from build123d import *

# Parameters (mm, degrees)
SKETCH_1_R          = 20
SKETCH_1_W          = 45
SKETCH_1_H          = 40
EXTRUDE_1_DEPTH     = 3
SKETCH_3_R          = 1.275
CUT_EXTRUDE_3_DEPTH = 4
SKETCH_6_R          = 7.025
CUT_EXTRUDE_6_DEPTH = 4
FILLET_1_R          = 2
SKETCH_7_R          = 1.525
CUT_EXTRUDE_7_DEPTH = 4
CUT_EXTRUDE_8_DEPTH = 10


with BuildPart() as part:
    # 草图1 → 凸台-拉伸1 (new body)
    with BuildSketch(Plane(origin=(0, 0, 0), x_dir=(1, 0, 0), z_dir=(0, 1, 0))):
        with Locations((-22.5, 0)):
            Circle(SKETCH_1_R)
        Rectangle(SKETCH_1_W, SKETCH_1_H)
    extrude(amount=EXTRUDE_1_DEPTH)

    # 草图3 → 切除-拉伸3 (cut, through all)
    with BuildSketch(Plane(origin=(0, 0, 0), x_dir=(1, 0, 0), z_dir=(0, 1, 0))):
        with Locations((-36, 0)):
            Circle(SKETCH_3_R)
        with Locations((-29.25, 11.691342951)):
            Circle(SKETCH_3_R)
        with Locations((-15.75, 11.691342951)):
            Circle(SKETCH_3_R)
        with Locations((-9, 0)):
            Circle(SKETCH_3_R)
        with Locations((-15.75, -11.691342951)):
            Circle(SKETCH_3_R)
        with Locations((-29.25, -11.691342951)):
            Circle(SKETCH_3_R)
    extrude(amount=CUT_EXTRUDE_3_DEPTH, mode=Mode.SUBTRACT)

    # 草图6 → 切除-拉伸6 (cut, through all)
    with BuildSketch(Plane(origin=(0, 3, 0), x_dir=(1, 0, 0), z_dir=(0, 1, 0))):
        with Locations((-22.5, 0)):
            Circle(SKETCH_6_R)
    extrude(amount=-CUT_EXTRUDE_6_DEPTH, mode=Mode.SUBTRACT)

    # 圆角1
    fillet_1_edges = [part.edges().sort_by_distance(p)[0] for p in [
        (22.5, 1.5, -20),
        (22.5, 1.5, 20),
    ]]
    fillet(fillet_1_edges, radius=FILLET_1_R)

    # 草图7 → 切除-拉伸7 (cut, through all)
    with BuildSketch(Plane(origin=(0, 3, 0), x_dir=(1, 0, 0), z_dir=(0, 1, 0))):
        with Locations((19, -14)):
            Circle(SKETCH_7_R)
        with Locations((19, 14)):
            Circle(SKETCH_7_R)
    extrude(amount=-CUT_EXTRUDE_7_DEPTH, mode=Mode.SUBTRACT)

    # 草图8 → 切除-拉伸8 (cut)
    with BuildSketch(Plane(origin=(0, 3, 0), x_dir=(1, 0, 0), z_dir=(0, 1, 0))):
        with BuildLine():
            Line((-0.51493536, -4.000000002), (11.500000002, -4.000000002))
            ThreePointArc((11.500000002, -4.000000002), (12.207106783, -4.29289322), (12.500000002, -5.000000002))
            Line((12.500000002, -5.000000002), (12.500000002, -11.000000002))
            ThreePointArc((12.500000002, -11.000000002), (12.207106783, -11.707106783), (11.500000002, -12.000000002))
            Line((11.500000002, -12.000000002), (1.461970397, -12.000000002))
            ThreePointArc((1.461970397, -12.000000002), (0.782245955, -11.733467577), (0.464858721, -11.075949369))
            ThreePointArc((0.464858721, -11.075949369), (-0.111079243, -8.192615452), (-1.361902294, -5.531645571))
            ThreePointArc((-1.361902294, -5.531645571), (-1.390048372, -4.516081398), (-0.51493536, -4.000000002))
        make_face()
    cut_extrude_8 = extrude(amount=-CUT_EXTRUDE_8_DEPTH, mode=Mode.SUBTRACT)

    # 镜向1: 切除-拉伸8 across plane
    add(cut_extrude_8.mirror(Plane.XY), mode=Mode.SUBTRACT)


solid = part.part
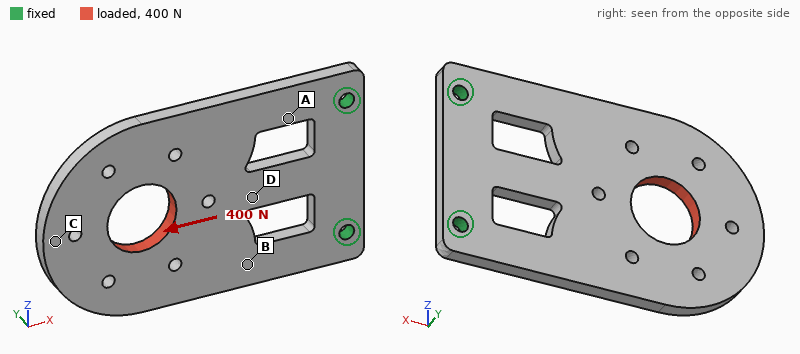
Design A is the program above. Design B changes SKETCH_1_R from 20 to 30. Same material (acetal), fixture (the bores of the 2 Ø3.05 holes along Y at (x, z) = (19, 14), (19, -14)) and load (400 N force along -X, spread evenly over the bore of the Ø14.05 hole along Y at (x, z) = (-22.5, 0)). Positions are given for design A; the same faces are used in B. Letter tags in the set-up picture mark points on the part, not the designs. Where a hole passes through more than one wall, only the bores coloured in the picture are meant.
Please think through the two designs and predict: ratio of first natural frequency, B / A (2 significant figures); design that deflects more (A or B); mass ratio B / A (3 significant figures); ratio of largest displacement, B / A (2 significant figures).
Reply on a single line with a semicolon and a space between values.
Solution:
0.62; A; 1.54; 0.88
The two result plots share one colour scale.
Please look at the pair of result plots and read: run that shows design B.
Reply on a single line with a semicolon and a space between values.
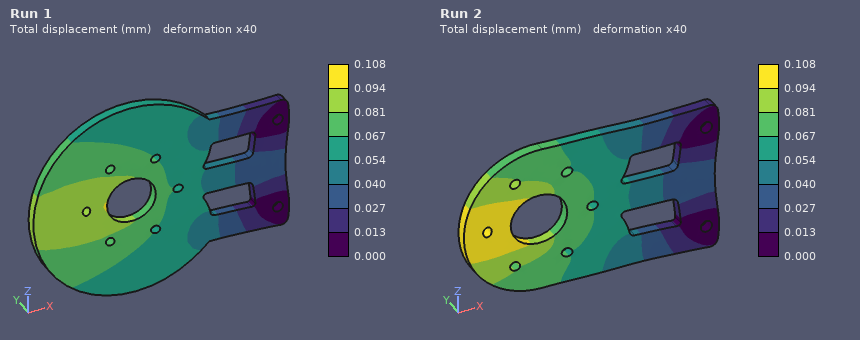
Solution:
Run 1
